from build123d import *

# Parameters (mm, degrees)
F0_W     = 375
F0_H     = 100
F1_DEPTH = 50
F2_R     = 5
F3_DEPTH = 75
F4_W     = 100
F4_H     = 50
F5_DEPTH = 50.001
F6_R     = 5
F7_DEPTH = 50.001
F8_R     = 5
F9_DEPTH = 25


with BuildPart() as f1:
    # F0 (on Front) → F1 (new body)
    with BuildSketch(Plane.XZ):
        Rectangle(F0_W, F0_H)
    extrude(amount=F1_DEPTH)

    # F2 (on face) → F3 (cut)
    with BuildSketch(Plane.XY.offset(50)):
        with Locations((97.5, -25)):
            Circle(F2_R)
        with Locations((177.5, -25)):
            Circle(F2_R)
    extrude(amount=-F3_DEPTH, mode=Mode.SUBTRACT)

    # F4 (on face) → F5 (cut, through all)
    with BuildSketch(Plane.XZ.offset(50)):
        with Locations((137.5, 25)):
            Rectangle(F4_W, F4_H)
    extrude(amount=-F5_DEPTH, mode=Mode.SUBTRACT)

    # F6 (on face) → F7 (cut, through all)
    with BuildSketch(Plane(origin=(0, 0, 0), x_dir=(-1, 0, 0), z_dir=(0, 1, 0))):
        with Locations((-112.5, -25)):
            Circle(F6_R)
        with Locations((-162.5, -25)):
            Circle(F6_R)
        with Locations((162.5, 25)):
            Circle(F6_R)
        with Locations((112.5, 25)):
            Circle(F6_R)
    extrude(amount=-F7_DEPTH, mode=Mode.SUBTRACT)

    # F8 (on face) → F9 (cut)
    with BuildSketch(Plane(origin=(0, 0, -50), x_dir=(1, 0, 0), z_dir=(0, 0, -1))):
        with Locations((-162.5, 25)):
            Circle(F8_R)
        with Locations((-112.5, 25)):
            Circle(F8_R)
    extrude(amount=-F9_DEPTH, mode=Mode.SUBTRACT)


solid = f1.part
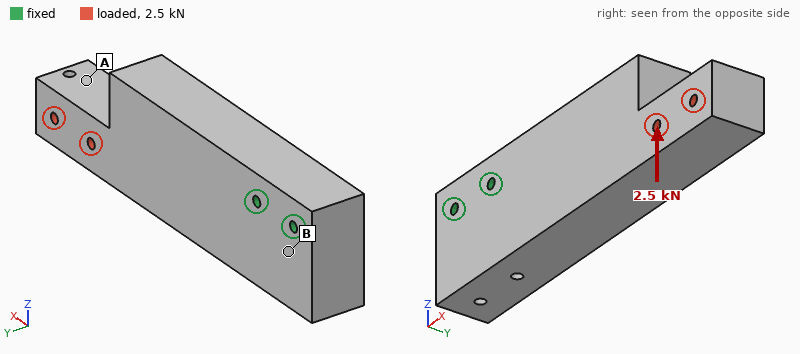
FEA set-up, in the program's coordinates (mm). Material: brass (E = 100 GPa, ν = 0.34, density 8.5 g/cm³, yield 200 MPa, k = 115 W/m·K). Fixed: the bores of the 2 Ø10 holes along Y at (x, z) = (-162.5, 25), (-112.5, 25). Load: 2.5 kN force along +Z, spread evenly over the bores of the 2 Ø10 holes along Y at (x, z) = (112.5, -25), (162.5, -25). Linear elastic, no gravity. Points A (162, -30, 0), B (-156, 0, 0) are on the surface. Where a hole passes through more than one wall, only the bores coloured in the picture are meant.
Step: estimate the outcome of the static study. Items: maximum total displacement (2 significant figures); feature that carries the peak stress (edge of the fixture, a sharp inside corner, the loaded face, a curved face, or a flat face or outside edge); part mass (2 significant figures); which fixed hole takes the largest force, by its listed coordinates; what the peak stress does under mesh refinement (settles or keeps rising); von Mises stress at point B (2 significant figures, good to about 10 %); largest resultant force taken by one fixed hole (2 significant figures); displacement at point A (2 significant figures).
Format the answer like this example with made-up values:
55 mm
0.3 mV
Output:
97 µm
edge of the fixture
14 kg
(-112.5, 25)
keeps rising
5.5 MPa
13 kN
83 µm
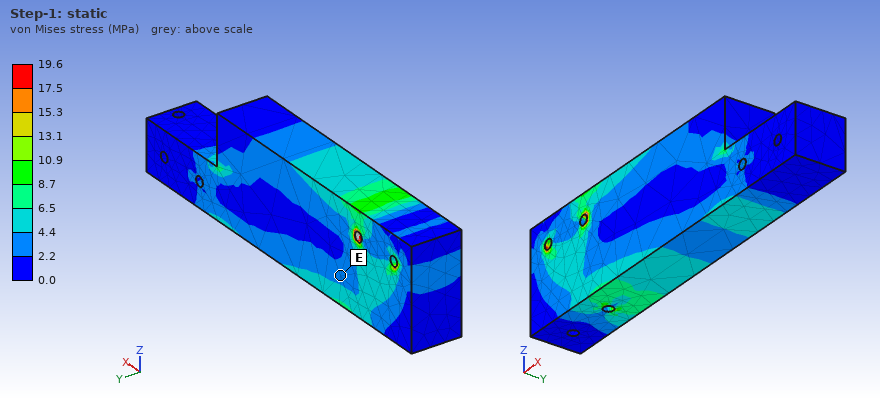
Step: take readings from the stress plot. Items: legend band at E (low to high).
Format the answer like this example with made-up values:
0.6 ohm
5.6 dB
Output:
2.2 to 4.4 MPa
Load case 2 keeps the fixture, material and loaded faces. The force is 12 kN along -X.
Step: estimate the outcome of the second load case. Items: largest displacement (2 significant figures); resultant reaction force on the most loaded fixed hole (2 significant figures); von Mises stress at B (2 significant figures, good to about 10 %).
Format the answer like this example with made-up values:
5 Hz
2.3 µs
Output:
68 µm
12 kN
5.5 MPa
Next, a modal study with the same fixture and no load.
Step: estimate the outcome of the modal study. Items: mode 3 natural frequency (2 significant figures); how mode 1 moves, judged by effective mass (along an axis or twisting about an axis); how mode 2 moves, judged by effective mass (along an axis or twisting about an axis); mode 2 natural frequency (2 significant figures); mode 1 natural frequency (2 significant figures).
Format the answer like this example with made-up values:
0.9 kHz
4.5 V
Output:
1500 Hz
along Y
along Z
500 Hz
340 Hz
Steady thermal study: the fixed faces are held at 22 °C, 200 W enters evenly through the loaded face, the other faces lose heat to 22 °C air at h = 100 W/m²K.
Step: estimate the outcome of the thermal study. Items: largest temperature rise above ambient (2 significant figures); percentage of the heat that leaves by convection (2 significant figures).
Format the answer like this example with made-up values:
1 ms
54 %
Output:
48 K
81 %
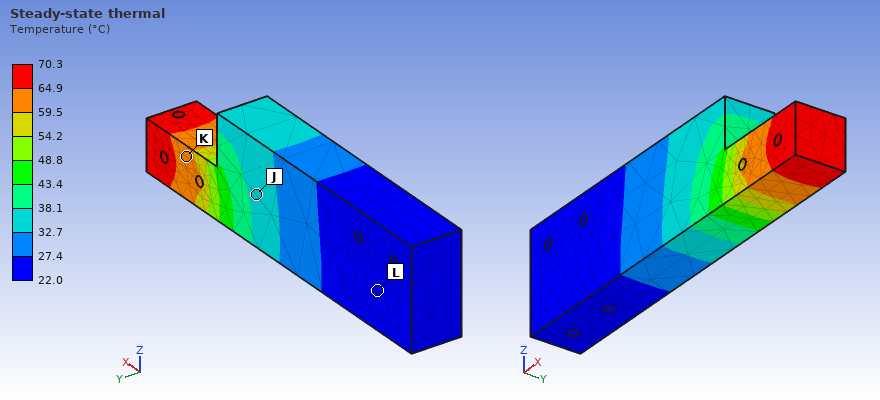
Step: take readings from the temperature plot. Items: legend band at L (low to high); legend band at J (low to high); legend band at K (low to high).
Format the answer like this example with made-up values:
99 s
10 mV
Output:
22.0 to 27.4 °C
32.7 to 38.1 °C
59.5 to 64.9 °C
